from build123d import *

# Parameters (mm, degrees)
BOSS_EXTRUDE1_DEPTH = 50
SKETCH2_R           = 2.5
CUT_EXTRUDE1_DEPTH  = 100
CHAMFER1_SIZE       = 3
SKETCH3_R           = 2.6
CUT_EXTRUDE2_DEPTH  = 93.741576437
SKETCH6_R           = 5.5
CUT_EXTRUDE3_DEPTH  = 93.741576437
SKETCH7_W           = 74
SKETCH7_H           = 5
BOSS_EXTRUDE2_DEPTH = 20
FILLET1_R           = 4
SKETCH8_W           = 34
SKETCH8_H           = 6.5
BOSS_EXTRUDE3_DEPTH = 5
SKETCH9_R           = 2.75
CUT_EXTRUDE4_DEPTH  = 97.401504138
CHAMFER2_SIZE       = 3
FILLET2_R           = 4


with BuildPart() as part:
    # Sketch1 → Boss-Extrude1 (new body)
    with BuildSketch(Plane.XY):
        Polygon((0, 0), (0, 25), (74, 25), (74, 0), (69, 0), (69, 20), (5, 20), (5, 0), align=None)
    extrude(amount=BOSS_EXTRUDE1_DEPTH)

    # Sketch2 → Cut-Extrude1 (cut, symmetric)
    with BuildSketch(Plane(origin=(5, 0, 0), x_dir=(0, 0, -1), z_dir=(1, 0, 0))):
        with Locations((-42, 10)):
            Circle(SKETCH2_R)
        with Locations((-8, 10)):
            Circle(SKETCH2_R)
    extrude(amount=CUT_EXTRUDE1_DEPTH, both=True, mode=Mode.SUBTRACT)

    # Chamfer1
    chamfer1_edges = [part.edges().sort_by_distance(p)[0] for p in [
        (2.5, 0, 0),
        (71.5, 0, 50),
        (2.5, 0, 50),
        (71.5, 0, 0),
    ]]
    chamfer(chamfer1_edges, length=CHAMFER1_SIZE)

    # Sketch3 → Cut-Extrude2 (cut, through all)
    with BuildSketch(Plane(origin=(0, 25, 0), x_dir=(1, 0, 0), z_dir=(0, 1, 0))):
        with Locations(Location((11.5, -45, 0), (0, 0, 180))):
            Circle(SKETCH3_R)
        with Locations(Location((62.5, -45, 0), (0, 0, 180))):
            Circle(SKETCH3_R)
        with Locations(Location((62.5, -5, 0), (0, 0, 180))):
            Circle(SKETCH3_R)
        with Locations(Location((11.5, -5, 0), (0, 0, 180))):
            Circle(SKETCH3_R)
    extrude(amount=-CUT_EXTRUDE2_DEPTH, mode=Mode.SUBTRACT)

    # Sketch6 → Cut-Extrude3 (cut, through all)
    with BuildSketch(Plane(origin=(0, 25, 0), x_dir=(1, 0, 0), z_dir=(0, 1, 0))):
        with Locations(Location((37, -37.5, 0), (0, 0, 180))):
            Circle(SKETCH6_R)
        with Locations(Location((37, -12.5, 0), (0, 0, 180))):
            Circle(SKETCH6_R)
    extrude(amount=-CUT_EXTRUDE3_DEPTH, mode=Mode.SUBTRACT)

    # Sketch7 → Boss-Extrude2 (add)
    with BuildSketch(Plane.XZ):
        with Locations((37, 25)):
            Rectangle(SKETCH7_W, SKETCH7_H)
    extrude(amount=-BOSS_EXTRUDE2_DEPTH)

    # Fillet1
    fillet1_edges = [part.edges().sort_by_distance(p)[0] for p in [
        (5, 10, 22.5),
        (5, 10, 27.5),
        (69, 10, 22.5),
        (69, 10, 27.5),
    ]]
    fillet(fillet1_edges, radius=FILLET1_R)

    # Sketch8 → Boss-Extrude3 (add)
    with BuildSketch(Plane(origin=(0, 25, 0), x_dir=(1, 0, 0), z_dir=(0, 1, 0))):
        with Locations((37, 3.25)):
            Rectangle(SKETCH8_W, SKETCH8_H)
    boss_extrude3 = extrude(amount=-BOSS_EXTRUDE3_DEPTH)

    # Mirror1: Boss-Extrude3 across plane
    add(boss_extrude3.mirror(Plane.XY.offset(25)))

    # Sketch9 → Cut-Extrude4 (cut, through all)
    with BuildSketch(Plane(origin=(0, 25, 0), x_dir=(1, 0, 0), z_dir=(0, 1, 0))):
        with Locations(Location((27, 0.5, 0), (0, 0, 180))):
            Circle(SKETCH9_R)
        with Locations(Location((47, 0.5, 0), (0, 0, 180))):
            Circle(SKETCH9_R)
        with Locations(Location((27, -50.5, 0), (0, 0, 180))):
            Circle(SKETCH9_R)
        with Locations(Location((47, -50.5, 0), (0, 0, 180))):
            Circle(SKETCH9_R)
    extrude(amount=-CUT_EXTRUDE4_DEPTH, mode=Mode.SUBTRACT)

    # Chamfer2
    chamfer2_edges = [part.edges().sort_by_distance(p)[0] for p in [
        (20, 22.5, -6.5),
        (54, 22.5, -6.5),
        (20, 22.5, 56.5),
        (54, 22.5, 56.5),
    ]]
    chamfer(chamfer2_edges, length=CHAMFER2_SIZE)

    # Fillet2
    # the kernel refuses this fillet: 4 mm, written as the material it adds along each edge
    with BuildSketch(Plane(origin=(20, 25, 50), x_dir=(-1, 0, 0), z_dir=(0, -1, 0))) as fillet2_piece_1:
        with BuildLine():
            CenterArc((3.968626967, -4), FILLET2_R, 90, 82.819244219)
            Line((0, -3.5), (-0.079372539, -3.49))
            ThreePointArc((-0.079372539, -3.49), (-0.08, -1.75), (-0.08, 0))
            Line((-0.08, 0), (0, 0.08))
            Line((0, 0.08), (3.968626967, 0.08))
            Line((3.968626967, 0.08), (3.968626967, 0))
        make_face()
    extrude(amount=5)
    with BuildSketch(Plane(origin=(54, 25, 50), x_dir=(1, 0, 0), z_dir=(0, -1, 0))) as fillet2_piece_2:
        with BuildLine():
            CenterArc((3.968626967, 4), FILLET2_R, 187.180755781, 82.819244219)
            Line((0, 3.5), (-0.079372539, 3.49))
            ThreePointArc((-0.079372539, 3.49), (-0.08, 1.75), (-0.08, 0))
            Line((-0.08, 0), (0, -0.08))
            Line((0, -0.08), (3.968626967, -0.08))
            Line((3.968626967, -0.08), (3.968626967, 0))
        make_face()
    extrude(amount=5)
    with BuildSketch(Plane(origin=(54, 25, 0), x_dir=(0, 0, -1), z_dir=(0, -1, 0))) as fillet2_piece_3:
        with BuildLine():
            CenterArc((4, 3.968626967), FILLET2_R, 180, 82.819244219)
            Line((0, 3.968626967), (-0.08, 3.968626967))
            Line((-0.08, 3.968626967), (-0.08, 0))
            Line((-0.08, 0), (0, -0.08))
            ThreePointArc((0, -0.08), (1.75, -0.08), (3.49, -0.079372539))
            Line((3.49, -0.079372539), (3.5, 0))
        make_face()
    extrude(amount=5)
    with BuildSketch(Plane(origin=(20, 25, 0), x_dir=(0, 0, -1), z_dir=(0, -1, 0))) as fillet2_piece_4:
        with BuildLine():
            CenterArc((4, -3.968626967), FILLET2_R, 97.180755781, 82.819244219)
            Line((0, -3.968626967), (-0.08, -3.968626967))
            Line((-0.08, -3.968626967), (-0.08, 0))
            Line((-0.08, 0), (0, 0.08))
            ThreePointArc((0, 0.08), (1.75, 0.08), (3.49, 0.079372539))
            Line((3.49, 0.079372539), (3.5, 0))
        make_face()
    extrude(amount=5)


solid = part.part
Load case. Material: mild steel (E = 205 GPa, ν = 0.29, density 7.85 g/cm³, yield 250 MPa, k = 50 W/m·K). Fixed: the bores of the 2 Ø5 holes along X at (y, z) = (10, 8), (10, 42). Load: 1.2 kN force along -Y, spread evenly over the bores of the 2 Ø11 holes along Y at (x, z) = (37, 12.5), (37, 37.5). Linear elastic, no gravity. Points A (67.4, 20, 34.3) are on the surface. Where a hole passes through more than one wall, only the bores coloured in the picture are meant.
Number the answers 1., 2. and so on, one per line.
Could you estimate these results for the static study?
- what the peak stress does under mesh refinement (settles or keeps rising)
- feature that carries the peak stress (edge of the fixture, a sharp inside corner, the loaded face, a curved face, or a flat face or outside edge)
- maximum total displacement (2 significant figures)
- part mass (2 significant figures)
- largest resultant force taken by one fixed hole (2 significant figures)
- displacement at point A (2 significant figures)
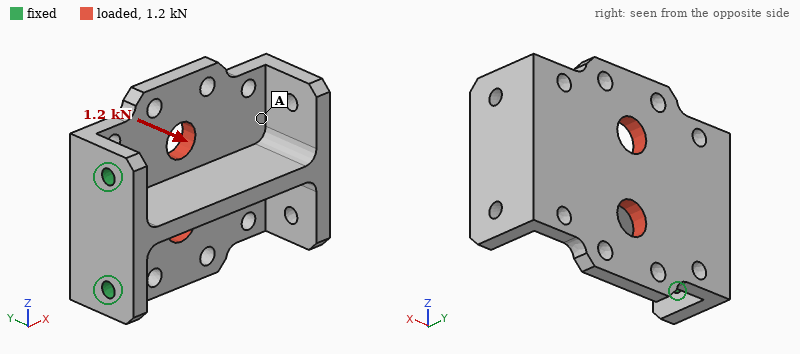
1. keeps rising
2. edge of the fixture
3. 0.17 mm
4. 270 g
5. 670 N
6. 0.15 mm
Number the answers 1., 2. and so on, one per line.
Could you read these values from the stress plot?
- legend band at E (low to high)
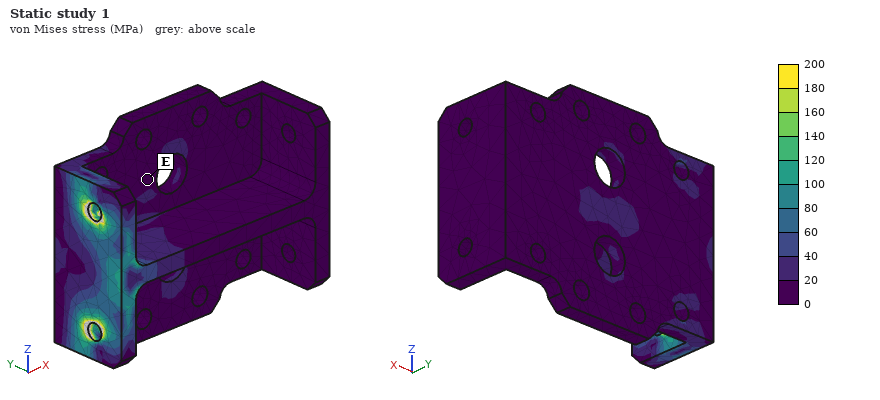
1. 0 to 20 MPa
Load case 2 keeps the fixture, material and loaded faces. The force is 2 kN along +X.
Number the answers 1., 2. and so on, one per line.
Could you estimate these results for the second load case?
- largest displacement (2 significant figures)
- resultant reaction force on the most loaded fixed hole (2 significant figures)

1. 74 µm
2. 1.0 kN
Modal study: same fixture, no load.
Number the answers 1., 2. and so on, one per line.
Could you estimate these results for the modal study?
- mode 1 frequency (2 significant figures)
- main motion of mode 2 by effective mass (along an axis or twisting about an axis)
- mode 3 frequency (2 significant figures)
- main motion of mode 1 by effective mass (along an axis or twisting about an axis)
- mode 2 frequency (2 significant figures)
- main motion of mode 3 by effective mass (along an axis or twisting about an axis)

1. 920 Hz
2. along Z
3. 2400 Hz
4. along Y
5. 1500 Hz
6. along Z
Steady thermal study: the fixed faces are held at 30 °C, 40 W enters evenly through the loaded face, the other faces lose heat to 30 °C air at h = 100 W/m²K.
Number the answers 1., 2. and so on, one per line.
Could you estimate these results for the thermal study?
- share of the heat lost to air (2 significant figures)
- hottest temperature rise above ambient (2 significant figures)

1. 77 %
2. 42 K
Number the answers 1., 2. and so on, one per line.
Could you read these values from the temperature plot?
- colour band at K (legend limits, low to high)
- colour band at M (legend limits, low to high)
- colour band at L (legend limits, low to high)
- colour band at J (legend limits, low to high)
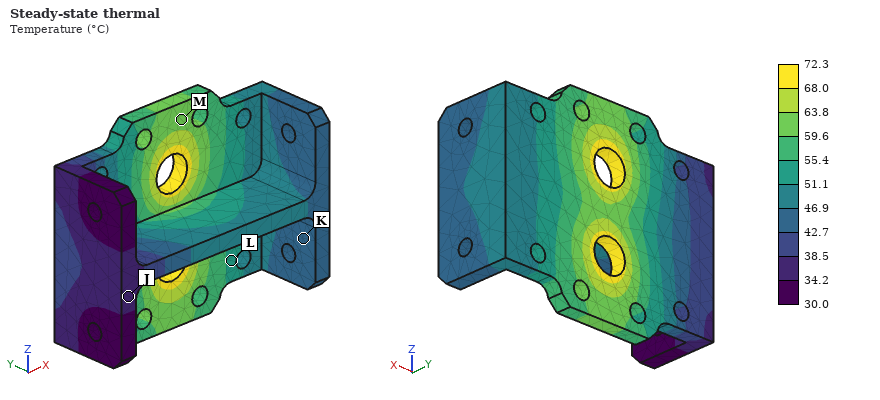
1. 42.7 to 46.9 °C
2. 59.6 to 63.8 °C
3. 51.1 to 55.4 °C
4. 34.2 to 38.5 °C
